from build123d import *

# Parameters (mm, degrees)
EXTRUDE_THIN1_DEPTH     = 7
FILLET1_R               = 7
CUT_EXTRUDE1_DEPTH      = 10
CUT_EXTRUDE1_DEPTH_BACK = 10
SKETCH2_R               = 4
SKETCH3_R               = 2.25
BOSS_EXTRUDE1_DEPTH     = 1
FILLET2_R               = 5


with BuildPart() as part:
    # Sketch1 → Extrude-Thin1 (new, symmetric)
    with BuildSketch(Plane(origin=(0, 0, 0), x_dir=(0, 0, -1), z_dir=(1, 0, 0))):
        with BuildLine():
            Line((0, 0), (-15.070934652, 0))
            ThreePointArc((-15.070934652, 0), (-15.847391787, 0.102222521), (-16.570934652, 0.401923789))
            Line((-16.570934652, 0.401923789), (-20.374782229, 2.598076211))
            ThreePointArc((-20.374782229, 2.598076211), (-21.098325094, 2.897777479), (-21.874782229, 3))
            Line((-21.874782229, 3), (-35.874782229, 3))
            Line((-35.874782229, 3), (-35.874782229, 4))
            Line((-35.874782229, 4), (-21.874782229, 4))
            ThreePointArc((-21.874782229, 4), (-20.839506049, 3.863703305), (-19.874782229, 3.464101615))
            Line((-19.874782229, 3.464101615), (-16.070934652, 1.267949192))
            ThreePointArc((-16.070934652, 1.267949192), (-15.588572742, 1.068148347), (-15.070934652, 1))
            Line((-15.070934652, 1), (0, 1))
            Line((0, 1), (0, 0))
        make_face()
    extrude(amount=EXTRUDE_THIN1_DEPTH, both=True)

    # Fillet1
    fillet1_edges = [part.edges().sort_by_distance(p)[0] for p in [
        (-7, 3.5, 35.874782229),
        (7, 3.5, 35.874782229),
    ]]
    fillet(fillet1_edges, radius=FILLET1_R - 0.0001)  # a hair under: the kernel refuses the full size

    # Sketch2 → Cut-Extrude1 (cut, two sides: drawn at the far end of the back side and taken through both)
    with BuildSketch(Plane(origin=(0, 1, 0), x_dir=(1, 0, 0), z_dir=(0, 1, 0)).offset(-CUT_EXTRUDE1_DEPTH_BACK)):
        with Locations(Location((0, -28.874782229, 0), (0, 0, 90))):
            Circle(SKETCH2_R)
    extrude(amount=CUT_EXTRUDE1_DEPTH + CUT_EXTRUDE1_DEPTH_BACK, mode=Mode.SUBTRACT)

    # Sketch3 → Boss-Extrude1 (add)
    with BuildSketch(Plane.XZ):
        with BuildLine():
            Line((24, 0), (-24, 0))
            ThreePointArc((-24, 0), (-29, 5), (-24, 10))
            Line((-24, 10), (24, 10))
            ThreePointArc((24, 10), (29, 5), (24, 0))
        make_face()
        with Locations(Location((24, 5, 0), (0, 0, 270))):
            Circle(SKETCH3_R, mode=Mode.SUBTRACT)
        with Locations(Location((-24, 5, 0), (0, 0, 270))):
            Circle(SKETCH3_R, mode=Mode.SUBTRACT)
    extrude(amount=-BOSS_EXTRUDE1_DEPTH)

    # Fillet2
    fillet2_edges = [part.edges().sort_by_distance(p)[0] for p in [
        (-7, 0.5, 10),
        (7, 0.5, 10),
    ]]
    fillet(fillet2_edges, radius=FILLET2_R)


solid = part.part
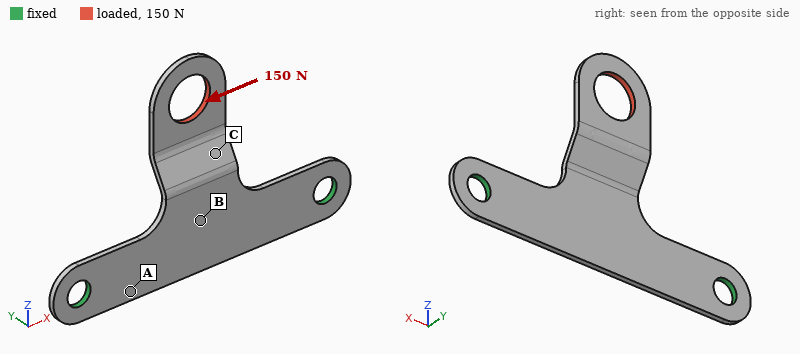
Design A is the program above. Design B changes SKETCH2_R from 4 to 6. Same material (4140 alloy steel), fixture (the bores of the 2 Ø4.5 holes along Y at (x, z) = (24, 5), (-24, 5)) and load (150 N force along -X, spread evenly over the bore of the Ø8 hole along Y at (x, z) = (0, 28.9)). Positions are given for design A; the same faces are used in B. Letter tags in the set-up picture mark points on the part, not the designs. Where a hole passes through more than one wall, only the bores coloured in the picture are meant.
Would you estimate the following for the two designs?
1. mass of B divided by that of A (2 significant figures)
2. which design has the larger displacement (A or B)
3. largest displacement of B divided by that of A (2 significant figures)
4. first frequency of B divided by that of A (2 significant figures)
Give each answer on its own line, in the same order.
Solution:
0.93
B
2.1
1.3
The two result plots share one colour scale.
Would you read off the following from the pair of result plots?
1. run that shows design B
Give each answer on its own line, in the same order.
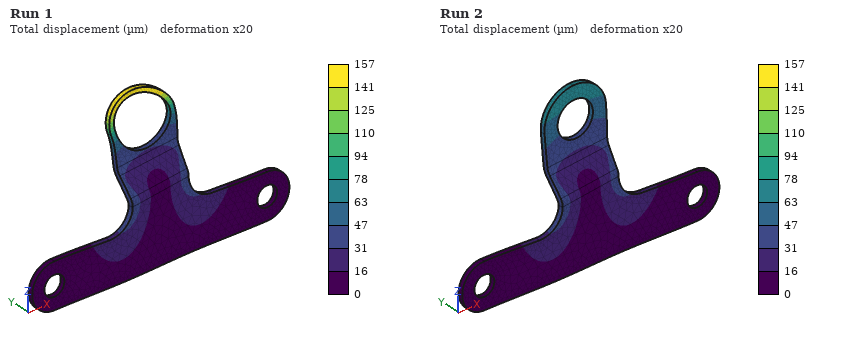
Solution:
Run 1
